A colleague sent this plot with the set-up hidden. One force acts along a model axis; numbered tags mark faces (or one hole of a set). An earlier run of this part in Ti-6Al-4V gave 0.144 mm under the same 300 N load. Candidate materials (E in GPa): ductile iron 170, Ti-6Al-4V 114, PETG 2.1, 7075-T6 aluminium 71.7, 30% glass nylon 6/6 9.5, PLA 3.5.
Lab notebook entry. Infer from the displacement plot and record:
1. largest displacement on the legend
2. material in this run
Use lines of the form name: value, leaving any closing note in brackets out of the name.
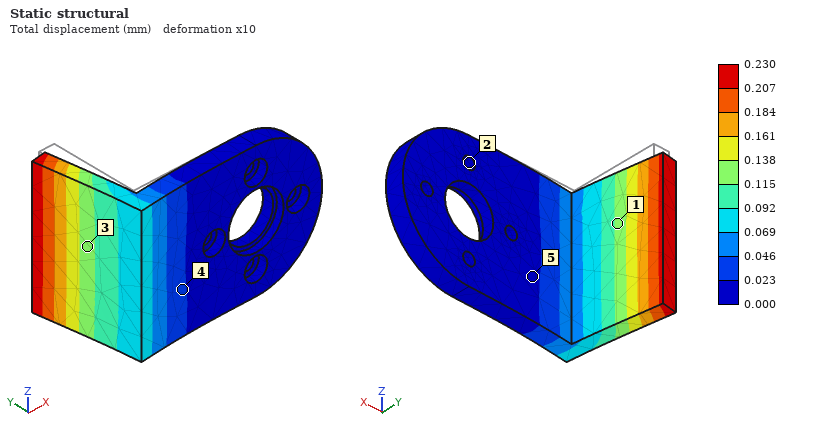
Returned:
largest displacement on the legend: 0.230 mm
material in this run: 7075-T6 aluminium
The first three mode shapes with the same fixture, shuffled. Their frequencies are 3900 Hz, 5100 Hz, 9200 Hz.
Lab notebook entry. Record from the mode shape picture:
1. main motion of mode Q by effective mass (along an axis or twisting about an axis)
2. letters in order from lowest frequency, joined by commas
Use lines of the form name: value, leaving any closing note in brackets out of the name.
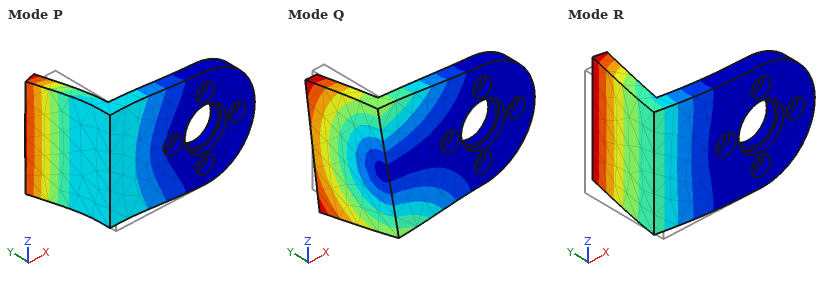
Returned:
main motion of mode Q by effective mass: along Z
letters in order from lowest frequency, joined by commas: R, Q, P
